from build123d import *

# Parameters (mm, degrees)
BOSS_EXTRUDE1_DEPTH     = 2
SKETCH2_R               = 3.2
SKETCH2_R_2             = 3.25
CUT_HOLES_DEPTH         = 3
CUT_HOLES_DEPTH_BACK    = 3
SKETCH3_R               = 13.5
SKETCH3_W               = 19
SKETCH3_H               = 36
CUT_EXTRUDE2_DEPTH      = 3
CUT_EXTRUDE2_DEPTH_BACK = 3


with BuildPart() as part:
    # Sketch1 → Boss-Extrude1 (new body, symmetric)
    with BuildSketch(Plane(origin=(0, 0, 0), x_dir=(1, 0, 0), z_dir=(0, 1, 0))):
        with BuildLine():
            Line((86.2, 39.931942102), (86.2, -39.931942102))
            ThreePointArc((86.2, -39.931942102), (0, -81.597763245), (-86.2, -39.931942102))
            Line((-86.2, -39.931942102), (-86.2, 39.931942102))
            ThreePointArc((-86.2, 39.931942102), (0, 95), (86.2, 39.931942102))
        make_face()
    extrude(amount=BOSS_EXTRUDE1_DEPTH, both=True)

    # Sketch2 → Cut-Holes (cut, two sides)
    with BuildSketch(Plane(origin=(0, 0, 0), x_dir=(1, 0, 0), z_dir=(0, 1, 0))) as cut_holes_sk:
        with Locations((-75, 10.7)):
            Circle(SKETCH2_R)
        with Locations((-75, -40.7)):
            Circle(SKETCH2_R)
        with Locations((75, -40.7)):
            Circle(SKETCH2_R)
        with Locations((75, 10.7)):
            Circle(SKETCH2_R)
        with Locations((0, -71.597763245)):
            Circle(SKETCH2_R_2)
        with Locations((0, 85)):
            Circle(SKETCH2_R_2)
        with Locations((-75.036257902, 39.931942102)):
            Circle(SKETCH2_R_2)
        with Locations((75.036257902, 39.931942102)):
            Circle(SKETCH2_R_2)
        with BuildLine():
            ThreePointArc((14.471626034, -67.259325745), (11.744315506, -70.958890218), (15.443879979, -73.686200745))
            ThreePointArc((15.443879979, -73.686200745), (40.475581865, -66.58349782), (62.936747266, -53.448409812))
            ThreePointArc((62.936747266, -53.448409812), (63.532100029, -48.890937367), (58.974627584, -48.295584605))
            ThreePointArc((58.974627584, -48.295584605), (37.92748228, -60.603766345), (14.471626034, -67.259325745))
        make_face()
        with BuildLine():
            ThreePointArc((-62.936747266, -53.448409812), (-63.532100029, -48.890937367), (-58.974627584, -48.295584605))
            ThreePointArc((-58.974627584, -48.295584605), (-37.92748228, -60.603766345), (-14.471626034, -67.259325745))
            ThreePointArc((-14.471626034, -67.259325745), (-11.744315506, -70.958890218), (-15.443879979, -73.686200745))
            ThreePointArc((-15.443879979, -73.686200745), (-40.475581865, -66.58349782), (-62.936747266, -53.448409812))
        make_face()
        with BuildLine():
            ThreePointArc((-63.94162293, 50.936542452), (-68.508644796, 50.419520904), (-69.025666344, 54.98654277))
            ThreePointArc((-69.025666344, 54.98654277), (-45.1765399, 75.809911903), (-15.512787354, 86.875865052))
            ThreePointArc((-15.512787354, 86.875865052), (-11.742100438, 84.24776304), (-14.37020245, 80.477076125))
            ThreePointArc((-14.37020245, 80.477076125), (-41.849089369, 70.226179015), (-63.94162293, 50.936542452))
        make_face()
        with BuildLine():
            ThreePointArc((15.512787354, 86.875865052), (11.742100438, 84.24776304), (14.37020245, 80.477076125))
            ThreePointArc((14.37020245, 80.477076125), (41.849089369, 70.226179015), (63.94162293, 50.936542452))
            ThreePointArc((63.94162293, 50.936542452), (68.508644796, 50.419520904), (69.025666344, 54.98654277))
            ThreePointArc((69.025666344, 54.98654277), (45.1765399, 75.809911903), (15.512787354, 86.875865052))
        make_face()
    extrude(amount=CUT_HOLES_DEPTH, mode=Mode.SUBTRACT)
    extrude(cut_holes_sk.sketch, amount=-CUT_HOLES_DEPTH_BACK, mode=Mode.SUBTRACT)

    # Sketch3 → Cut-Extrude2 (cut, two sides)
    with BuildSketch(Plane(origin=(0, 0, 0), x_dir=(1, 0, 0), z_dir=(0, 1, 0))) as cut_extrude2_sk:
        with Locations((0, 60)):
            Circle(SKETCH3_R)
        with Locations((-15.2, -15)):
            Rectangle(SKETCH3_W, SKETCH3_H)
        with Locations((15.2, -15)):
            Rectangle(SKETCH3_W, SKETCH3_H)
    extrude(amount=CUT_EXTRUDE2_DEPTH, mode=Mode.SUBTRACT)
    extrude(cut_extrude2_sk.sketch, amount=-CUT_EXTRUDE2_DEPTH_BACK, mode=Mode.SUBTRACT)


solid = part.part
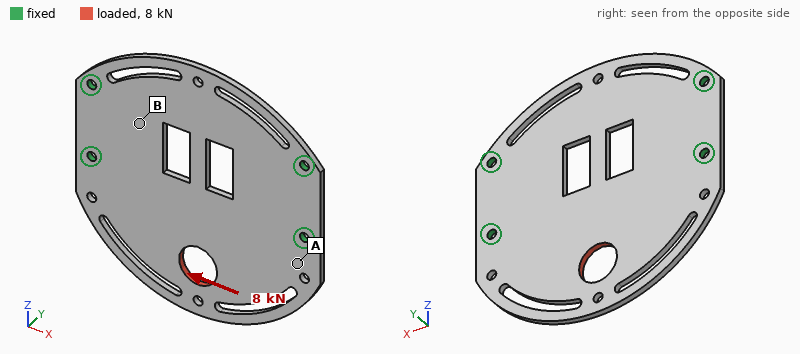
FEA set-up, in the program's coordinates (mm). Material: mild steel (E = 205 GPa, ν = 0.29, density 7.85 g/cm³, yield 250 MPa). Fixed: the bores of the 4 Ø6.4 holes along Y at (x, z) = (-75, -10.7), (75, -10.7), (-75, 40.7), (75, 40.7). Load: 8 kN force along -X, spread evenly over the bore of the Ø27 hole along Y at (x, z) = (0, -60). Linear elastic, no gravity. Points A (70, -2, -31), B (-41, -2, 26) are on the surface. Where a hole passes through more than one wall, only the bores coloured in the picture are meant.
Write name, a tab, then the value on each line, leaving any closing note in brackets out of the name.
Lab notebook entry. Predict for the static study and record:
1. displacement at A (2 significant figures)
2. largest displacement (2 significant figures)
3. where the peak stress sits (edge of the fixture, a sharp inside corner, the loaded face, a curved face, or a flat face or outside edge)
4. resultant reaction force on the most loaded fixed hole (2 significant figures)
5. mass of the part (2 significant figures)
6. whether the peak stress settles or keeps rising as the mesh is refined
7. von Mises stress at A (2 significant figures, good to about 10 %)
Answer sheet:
displacement at A	6.0 µm
largest displacement	21 µm
where the peak stress sits	edge of the fixture
resultant reaction force on the most loaded fixed hole	4.2 kN
mass of the part	680 g
whether the peak stress settles or keeps rising as the mesh is refined	keeps rising
von Mises stress at A	26 MPa
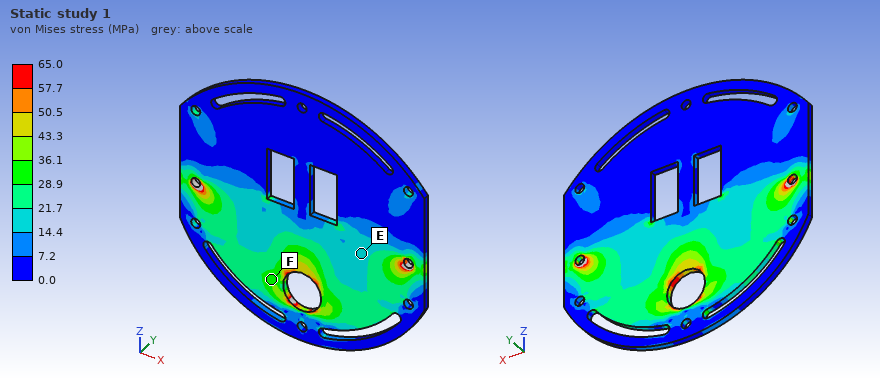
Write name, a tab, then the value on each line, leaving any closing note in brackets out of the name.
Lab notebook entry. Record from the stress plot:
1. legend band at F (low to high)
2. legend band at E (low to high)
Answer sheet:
legend band at F	28.9 to 36.1 MPa
legend band at E	14.4 to 21.7 MPa
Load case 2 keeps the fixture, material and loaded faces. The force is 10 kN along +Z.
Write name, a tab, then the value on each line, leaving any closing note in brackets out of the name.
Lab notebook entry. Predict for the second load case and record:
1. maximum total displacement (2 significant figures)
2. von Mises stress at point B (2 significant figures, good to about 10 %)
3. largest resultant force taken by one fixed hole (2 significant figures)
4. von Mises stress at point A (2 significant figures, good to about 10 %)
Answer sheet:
maximum total displacement	22 µm
von Mises stress at point B	17 MPa
largest resultant force taken by one fixed hole	3.3 kN
von Mises stress at point A	18 MPa
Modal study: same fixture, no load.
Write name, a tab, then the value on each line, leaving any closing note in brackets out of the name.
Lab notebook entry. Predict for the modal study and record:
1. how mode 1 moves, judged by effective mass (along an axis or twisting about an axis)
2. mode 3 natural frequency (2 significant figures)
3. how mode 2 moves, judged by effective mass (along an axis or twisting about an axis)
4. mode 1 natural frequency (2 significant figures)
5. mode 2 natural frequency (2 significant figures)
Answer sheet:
how mode 1 moves, judged by effective mass	along Y
mode 3 natural frequency	1100 Hz
how mode 2 moves, judged by effective mass	along Y
mode 1 natural frequency	460 Hz
mode 2 natural frequency	820 Hz
